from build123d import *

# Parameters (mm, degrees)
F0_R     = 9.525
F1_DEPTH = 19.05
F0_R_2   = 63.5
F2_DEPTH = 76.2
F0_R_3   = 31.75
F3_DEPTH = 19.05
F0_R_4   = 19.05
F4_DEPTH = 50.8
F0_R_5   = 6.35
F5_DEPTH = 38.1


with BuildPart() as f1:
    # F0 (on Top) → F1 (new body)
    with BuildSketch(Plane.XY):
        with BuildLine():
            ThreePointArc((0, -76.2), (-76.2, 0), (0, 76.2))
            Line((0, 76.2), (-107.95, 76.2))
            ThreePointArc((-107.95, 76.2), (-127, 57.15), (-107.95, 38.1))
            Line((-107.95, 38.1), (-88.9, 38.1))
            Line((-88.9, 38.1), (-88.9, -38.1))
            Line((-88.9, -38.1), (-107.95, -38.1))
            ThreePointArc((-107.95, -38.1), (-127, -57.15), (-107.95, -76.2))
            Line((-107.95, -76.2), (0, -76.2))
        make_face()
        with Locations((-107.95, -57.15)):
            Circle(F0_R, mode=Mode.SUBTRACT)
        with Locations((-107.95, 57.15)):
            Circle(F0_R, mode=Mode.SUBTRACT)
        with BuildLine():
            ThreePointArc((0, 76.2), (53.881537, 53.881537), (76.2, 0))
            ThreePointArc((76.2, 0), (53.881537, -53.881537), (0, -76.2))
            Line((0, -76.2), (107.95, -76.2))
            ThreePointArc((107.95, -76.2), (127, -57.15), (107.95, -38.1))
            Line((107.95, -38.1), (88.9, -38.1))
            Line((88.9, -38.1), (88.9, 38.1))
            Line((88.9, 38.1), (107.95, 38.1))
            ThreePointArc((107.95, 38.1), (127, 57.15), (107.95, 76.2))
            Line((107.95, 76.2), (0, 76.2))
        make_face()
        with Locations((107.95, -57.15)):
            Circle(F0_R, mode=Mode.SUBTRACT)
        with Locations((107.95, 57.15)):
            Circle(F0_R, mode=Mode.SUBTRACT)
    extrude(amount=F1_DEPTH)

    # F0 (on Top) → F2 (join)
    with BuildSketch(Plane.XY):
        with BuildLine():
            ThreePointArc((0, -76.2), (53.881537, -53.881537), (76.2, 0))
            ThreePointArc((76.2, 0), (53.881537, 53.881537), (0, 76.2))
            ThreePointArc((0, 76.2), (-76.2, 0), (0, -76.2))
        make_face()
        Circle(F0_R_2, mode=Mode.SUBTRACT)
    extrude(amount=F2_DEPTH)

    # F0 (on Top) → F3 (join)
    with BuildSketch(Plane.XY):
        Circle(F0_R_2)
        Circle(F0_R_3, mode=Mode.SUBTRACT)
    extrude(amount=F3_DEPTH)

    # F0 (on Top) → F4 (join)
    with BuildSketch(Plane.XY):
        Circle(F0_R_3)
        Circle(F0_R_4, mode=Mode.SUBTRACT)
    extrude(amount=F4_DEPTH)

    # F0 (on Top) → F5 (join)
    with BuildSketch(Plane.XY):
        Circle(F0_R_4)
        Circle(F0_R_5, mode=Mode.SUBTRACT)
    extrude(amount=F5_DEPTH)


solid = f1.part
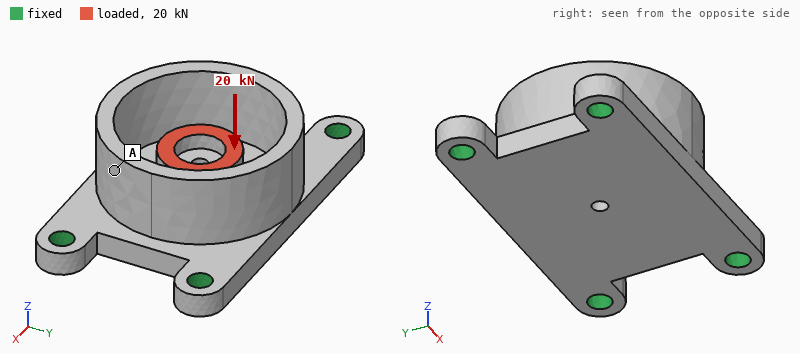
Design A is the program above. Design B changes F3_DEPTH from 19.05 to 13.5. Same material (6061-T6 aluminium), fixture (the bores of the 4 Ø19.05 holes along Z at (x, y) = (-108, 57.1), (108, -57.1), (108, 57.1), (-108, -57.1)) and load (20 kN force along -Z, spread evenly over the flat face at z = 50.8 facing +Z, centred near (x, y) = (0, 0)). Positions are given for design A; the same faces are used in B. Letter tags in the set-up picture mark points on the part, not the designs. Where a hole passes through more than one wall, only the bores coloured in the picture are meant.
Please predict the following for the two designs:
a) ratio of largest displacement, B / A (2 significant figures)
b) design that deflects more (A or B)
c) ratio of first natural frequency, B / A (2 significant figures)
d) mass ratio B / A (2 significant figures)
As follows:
1.3
B
0.98
0.95
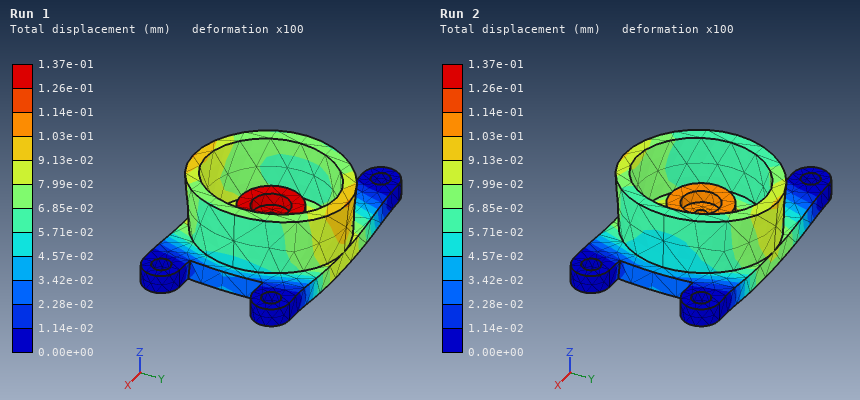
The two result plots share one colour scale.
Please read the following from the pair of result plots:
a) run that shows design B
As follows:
Run 1
